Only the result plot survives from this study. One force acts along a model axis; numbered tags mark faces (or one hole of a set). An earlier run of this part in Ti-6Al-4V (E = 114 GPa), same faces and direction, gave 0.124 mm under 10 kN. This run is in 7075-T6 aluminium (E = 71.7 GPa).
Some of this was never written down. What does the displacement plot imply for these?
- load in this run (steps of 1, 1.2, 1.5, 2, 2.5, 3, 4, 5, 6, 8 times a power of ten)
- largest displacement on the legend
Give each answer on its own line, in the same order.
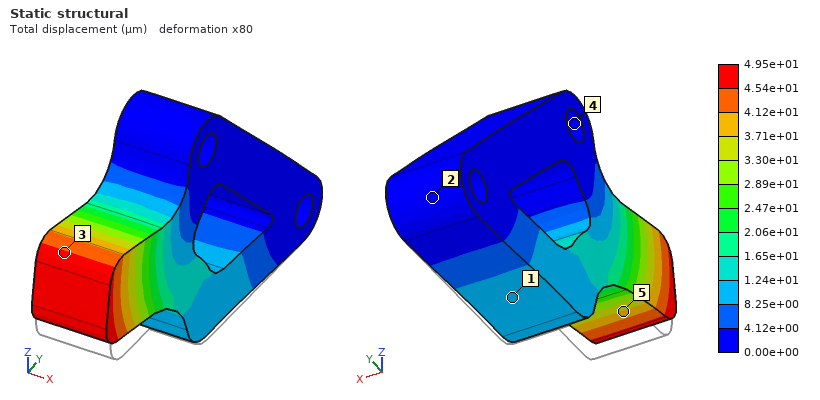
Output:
2.5 kN
4.95e+01 µm
